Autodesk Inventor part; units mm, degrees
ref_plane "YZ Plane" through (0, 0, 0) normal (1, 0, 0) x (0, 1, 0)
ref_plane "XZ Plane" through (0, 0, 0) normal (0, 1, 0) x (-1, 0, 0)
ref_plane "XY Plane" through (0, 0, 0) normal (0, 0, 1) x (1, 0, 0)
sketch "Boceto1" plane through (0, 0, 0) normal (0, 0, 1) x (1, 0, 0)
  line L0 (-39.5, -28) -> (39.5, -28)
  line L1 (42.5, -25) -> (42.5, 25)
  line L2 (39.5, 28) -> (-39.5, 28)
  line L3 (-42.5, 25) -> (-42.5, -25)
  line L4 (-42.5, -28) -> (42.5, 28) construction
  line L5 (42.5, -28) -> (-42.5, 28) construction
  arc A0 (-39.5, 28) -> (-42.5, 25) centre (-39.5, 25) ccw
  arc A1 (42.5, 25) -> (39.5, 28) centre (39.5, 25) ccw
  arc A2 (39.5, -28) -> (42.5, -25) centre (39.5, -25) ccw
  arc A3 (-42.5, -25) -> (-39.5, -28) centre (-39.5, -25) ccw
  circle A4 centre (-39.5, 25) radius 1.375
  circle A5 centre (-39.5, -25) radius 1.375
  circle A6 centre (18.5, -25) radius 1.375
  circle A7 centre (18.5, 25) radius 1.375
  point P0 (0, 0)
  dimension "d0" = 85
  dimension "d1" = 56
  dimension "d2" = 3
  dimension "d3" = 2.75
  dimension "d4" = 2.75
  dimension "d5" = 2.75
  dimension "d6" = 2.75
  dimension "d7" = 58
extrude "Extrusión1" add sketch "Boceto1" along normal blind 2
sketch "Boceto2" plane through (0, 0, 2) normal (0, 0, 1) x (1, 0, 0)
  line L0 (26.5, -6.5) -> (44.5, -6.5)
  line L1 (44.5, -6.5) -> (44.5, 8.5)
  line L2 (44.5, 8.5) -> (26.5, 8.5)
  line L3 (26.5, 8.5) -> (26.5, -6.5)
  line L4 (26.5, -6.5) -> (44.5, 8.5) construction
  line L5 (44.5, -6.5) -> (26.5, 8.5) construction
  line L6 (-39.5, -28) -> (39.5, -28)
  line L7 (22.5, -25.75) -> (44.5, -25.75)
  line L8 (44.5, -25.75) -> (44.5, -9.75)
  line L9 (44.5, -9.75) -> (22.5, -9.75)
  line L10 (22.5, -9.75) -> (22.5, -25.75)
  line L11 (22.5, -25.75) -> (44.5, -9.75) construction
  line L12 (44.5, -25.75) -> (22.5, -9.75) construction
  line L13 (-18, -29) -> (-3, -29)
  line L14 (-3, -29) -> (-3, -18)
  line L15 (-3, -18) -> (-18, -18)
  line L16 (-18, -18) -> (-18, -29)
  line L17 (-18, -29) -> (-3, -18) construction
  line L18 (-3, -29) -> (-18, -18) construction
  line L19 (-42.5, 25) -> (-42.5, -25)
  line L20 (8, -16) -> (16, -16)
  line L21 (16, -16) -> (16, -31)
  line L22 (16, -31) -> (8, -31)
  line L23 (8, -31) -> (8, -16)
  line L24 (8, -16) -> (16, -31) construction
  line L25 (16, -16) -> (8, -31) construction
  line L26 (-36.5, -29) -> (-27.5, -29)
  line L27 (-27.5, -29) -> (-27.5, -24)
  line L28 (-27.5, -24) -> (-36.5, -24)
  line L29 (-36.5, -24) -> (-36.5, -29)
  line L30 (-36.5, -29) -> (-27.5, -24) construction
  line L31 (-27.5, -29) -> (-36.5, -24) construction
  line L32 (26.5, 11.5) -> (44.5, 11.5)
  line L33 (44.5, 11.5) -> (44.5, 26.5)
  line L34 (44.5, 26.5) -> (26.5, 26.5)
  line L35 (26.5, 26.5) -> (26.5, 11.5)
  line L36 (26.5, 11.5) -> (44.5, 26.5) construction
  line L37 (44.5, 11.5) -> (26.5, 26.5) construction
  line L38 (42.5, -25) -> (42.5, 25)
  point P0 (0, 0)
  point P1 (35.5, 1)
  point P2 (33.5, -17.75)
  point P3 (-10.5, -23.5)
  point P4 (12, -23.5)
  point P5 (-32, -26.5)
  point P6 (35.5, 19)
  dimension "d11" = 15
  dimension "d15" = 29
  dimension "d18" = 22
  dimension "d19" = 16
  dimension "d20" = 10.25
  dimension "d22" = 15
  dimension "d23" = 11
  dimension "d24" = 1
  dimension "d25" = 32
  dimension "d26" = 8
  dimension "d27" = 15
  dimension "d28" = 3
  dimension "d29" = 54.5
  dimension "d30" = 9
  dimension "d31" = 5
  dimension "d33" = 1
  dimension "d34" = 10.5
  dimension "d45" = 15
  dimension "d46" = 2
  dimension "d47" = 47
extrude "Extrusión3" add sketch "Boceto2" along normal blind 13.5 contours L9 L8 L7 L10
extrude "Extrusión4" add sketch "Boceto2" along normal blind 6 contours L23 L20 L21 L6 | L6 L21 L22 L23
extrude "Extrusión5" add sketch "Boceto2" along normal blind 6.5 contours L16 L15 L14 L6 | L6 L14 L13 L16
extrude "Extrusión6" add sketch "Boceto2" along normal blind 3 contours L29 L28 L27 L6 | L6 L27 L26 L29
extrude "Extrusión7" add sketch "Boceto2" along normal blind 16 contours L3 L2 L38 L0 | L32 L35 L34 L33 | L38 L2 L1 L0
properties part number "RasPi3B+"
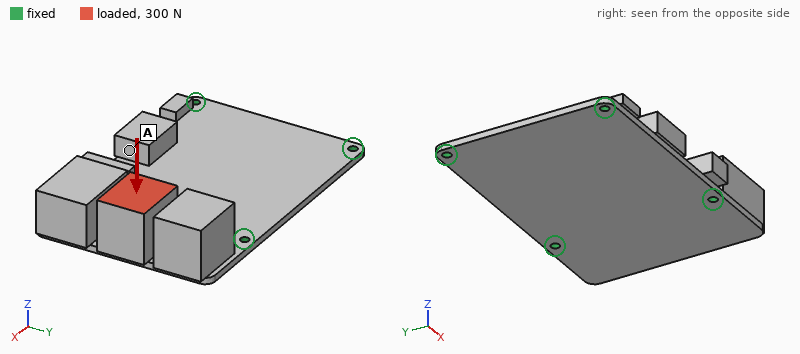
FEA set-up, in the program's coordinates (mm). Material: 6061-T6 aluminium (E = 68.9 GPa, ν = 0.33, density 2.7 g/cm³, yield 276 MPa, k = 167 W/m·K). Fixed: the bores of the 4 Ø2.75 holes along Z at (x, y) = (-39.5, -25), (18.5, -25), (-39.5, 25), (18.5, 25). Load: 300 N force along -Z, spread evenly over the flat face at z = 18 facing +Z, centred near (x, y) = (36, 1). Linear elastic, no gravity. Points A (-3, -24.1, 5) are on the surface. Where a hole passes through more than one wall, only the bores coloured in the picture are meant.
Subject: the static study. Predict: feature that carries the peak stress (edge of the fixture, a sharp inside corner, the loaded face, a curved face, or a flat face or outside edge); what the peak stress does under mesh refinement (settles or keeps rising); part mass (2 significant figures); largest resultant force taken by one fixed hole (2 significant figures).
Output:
edge of the fixture
keeps rising
67 g
170 N
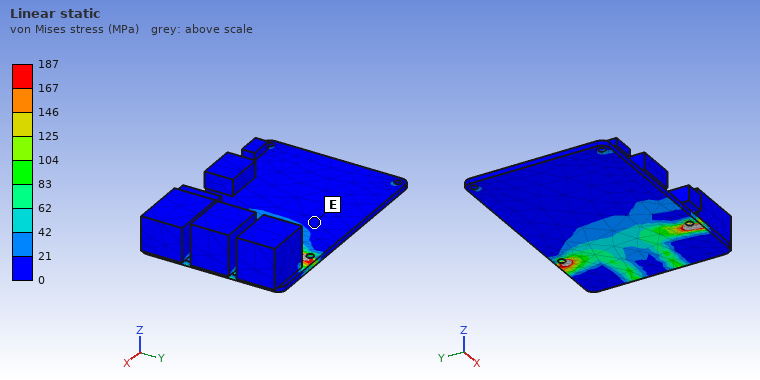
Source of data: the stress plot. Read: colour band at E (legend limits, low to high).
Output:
0 to 21 MPa
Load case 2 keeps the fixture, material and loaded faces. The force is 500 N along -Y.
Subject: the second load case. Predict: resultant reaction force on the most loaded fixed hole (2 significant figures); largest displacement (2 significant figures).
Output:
360 N
0.16 mm
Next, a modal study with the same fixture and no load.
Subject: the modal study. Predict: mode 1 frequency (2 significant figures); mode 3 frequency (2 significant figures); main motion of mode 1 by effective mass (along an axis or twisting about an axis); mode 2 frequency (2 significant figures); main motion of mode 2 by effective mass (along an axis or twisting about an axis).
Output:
710 Hz
2500 Hz
along Z
2200 Hz
along Z
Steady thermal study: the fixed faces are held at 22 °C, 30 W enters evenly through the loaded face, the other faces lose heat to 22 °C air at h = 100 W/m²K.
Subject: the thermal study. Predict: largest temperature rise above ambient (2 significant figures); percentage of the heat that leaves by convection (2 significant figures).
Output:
37 K
45 %
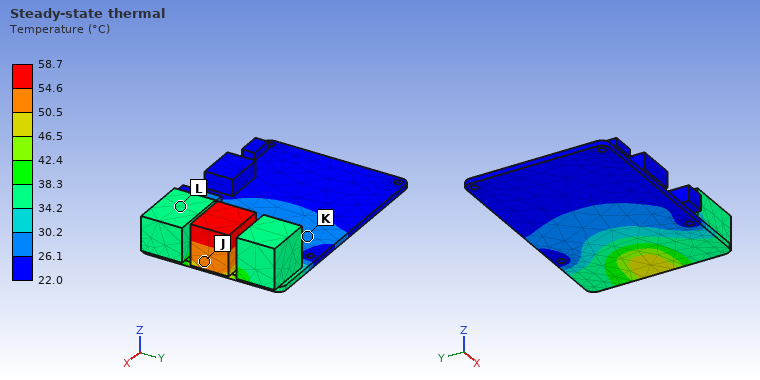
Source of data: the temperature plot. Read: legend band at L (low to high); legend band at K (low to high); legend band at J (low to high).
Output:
34.2 to 38.3 °C
26.1 to 30.2 °C
50.5 to 54.6 °C
